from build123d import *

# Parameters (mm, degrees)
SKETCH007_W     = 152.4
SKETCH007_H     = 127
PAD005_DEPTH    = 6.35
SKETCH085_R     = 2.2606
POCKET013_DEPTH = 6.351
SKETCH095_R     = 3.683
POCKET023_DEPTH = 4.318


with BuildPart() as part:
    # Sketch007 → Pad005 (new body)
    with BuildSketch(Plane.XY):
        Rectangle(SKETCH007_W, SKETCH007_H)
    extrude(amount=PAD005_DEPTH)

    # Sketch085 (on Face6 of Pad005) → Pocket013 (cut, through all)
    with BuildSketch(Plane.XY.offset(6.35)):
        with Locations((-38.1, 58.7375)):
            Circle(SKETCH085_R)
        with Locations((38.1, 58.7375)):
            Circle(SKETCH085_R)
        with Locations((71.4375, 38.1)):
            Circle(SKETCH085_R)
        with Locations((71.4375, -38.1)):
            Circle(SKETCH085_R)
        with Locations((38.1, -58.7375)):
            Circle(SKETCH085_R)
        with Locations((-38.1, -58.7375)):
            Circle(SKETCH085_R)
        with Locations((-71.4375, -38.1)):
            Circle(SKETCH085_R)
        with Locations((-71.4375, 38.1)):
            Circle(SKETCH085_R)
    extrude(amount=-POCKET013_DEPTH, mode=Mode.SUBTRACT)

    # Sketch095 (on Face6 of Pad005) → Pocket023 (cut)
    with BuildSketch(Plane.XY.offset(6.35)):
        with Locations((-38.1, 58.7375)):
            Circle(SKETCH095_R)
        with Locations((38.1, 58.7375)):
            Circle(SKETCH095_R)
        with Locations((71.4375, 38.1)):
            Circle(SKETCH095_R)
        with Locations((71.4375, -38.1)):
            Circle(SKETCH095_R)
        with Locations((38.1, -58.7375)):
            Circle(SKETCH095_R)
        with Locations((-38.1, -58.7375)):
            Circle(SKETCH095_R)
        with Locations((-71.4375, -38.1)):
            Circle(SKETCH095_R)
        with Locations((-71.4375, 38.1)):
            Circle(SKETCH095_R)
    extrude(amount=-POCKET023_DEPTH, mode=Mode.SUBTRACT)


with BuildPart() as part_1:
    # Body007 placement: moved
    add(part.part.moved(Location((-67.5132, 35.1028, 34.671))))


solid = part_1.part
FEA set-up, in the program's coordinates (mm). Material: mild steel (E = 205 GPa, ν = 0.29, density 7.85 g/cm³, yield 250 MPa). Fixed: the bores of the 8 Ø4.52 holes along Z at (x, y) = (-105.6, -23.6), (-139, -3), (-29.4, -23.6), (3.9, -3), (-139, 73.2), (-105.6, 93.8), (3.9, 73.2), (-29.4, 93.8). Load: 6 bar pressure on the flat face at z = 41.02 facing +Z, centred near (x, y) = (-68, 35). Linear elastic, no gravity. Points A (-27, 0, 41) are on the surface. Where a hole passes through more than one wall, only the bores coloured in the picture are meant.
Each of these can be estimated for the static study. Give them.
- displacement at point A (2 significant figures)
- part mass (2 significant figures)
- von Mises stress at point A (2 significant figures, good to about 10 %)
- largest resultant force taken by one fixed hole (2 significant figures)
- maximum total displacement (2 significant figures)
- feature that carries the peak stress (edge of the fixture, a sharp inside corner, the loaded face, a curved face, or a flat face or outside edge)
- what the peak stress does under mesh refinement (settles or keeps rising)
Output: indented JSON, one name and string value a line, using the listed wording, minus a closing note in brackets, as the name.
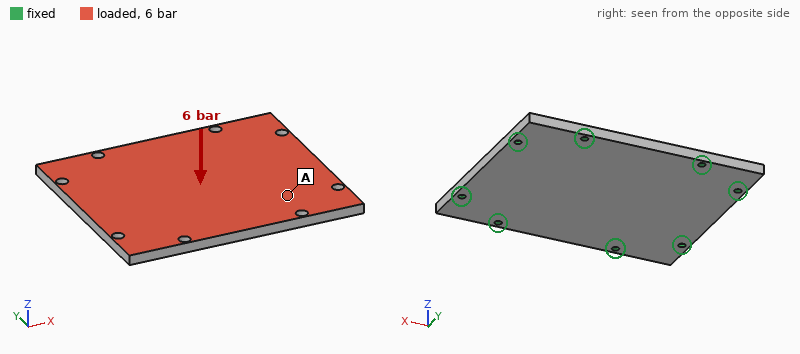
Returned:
{
  "displacement at point A": "0.052 mm",
  "part mass": "950 g",
  "von Mises stress at point A": "30 MPa",
  "largest resultant force taken by one fixed hole": "3.4 kN",
  "maximum total displacement": "0.13 mm",
  "feature that carries the peak stress": "edge of the fixture",
  "what the peak stress does under mesh refinement": "keeps rising"
}
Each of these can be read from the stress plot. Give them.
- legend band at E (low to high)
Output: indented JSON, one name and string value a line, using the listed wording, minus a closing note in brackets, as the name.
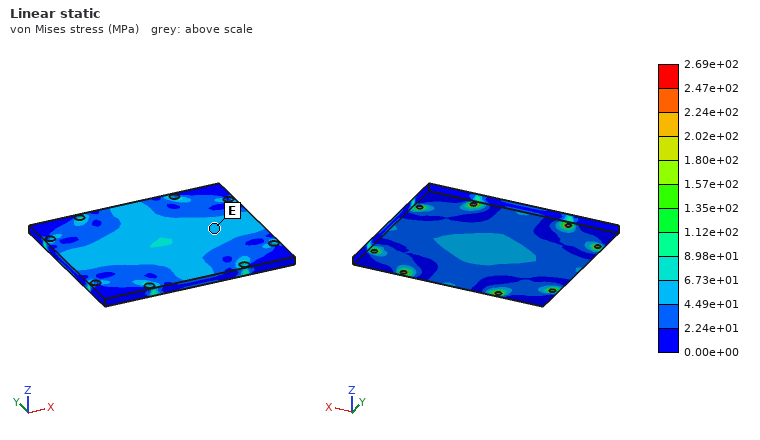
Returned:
{
  "legend band at E": "4.49e+01 to 6.73e+01 MPa"
}
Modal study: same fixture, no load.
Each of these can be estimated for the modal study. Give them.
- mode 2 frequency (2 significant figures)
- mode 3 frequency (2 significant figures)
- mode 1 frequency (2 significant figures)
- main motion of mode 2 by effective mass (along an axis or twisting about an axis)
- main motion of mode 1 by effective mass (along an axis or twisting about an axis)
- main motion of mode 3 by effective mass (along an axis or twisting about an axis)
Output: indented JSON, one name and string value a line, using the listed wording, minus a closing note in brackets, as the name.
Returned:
{
  "mode 2 frequency": "3400 Hz",
  "mode 3 frequency": "4000 Hz",
  "mode 1 frequency": "1800 Hz",
  "main motion of mode 2 by effective mass": "twisting about Y",
  "main motion of mode 1 by effective mass": "along Z",
  "main motion of mode 3 by effective mass": "twisting about X"
}
